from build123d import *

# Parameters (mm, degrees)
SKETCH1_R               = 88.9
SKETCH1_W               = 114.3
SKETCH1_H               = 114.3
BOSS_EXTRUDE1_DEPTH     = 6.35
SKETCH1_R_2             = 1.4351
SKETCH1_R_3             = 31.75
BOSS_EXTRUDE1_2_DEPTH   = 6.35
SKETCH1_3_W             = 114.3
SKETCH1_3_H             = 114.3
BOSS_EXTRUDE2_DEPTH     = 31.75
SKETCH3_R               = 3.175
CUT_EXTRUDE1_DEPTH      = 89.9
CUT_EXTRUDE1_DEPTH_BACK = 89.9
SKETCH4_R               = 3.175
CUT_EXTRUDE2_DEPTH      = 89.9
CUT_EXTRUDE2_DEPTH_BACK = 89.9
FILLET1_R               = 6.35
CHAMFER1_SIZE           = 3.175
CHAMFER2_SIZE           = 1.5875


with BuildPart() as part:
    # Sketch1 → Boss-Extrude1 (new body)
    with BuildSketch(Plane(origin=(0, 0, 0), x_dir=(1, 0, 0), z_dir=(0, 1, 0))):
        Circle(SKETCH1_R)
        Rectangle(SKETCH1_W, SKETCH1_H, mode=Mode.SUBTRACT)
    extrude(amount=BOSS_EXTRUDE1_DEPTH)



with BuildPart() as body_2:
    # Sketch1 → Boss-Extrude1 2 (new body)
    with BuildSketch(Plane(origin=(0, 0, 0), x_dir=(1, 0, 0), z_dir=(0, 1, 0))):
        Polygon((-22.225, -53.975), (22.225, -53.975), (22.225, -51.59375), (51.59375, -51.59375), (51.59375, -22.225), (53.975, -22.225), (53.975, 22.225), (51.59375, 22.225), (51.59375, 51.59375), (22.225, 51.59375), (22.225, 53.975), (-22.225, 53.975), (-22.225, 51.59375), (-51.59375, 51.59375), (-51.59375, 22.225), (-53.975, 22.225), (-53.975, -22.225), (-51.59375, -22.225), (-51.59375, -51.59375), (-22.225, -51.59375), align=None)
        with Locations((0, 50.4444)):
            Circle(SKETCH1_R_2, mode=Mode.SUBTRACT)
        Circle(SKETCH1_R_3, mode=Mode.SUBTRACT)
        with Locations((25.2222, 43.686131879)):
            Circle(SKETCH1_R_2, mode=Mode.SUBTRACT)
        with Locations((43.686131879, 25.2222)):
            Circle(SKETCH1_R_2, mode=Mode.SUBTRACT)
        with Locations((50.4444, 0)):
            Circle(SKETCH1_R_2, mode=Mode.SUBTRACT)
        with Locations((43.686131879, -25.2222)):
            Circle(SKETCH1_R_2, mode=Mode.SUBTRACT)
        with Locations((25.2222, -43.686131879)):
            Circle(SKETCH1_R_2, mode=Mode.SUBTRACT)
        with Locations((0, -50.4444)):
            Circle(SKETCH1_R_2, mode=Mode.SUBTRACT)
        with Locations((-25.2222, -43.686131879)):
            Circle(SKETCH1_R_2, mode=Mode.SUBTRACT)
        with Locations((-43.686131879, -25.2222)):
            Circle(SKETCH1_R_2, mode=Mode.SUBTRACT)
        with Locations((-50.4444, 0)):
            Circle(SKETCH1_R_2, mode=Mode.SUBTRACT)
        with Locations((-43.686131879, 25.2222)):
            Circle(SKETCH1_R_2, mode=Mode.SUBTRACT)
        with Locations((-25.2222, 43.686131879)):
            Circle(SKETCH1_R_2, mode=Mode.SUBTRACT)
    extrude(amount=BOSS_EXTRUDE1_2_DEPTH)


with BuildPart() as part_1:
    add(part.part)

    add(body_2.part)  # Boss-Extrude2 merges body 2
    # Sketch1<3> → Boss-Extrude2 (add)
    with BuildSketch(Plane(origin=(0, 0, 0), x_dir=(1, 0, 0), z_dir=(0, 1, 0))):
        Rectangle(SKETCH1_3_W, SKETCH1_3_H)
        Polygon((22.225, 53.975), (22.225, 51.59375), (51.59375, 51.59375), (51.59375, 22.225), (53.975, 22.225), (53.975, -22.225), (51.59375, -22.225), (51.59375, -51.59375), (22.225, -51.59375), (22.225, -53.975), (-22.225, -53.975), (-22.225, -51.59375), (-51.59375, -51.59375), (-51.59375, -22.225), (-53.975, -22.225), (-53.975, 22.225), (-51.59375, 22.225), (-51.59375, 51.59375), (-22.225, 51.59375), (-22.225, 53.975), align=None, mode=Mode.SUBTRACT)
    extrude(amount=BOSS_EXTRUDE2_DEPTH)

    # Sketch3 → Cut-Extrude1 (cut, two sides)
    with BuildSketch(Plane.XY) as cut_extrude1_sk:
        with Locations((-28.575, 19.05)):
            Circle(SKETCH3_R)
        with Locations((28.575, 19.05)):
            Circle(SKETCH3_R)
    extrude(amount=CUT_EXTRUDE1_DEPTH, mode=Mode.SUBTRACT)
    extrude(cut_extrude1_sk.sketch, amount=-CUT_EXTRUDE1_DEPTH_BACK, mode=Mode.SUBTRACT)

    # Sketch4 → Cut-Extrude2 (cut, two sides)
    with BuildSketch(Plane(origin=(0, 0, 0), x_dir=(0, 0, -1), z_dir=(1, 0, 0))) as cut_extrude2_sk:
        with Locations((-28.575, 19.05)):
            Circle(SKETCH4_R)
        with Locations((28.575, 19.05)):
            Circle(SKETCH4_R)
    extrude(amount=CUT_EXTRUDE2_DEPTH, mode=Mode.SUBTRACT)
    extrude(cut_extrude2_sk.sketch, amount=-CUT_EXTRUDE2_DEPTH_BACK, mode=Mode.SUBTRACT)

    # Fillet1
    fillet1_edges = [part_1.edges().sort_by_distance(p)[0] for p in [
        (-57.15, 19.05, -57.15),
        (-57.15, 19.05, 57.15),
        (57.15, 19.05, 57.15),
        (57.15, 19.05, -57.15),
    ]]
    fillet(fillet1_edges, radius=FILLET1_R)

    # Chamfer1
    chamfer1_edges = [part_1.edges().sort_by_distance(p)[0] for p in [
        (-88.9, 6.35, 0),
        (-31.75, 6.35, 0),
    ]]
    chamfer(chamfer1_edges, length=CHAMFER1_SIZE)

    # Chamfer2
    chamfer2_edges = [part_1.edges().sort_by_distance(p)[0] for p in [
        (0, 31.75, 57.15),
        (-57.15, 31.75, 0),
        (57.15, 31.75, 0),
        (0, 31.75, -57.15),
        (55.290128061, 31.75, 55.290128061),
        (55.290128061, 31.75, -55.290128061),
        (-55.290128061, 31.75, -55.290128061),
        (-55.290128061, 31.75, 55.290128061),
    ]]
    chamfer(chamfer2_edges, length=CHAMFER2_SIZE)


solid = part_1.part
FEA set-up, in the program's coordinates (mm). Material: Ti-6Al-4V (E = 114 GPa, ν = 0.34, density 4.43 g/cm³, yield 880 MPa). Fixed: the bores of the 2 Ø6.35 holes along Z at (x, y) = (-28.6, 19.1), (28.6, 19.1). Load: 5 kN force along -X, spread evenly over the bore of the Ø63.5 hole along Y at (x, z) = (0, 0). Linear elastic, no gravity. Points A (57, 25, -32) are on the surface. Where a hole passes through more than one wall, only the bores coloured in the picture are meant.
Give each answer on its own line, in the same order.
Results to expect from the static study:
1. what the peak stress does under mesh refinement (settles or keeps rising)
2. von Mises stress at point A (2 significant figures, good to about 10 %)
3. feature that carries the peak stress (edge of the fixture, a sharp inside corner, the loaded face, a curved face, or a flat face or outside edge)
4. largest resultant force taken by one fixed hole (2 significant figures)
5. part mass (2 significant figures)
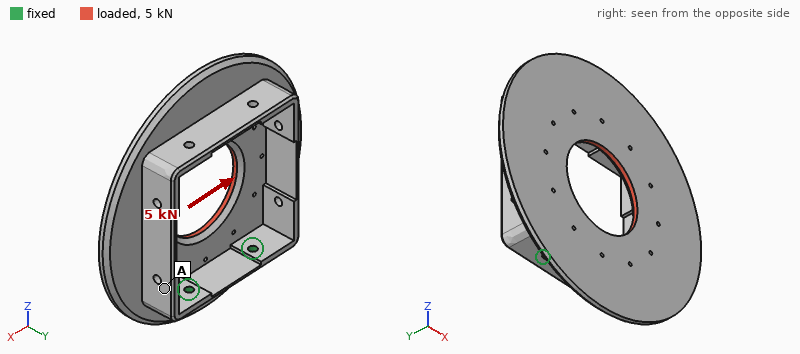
keeps rising
17 MPa
edge of the fixture
5.0 kN
800 g
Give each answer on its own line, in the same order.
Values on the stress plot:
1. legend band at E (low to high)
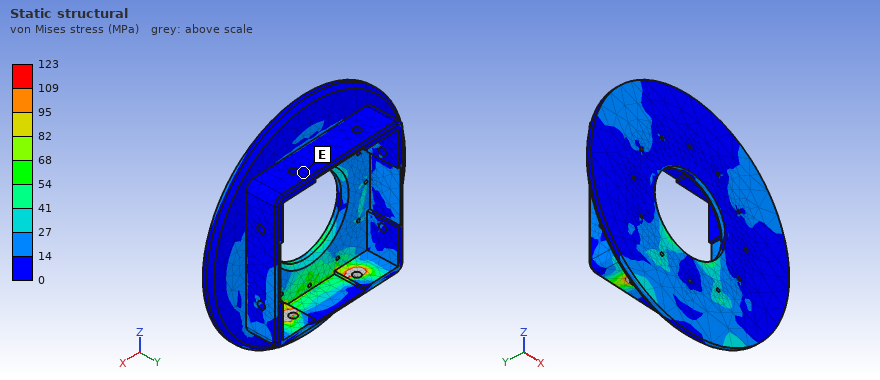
0 to 14 MPa
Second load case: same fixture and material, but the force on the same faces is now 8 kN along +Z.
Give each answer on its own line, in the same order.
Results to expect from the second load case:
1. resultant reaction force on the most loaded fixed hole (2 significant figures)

4.0 kN
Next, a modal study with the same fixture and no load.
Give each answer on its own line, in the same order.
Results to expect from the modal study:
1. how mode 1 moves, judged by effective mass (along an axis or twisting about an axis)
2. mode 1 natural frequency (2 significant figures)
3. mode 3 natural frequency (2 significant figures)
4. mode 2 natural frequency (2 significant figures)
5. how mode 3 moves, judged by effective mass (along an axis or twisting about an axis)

along Y
250 Hz
960 Hz
540 Hz
along X
